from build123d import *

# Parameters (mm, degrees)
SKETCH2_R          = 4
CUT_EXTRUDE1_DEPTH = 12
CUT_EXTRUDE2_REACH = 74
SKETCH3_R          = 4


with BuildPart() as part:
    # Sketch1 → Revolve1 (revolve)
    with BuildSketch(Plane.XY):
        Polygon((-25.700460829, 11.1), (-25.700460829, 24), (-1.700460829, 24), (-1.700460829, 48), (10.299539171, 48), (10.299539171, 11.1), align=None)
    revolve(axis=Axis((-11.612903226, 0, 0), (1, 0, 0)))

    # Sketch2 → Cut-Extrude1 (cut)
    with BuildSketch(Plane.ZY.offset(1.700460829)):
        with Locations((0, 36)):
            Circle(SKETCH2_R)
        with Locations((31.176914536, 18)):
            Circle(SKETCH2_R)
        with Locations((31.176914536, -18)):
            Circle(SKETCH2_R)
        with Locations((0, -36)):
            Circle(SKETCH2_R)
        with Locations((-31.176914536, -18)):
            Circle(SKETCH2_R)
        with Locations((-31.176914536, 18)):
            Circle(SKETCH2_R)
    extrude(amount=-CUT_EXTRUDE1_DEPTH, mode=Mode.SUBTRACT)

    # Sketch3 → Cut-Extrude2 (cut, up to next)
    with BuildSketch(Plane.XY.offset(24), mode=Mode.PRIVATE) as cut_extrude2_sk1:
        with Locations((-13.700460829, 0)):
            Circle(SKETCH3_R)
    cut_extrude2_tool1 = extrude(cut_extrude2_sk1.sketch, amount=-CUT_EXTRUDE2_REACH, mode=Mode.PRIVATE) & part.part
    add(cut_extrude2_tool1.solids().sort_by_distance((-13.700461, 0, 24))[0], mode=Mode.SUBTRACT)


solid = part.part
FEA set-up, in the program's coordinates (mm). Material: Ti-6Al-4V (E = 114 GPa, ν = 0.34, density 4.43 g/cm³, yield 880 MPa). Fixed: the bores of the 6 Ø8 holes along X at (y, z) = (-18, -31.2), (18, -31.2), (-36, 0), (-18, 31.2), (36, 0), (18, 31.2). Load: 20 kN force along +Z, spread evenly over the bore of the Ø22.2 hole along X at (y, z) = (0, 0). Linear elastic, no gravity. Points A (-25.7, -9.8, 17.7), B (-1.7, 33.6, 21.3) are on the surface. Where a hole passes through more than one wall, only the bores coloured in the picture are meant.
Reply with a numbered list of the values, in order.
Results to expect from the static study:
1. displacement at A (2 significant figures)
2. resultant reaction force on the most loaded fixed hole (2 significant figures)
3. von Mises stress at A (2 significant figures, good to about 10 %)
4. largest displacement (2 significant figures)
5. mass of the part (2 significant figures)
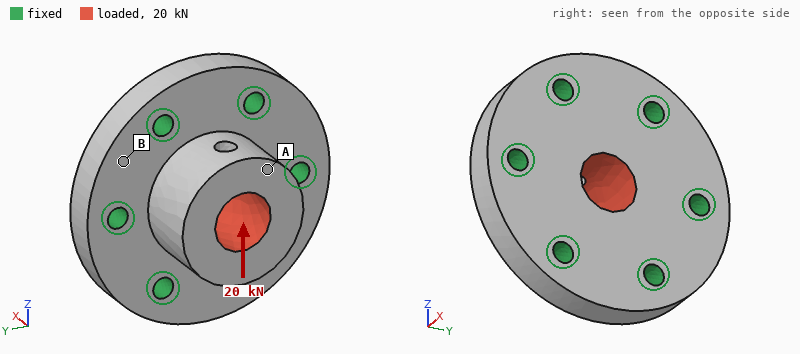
1. 12 µm
2. 4.9 kN
3. 11 MPa
4. 13 µm
5. 500 g
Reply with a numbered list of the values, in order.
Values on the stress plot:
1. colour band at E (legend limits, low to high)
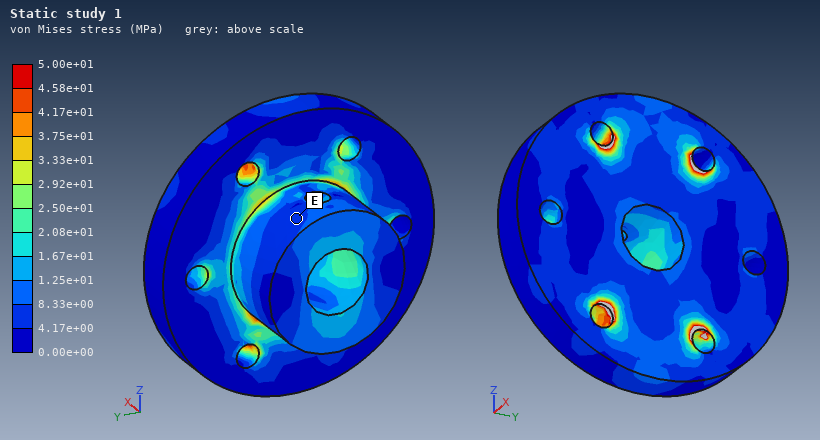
1. 4.17e+00 to 8.33e+00 MPa
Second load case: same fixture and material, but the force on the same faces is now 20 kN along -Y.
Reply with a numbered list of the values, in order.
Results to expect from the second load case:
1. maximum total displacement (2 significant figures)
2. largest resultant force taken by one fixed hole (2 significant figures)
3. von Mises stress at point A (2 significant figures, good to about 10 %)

1. 13 µm
2. 5.6 kN
3. 7.5 MPa
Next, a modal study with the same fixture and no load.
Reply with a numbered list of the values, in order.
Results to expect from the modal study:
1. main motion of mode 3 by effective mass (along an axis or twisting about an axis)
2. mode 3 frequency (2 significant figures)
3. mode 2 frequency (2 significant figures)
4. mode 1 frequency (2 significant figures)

1. along X
2. 16 kHz
3. 15 kHz
4. 15 kHz
